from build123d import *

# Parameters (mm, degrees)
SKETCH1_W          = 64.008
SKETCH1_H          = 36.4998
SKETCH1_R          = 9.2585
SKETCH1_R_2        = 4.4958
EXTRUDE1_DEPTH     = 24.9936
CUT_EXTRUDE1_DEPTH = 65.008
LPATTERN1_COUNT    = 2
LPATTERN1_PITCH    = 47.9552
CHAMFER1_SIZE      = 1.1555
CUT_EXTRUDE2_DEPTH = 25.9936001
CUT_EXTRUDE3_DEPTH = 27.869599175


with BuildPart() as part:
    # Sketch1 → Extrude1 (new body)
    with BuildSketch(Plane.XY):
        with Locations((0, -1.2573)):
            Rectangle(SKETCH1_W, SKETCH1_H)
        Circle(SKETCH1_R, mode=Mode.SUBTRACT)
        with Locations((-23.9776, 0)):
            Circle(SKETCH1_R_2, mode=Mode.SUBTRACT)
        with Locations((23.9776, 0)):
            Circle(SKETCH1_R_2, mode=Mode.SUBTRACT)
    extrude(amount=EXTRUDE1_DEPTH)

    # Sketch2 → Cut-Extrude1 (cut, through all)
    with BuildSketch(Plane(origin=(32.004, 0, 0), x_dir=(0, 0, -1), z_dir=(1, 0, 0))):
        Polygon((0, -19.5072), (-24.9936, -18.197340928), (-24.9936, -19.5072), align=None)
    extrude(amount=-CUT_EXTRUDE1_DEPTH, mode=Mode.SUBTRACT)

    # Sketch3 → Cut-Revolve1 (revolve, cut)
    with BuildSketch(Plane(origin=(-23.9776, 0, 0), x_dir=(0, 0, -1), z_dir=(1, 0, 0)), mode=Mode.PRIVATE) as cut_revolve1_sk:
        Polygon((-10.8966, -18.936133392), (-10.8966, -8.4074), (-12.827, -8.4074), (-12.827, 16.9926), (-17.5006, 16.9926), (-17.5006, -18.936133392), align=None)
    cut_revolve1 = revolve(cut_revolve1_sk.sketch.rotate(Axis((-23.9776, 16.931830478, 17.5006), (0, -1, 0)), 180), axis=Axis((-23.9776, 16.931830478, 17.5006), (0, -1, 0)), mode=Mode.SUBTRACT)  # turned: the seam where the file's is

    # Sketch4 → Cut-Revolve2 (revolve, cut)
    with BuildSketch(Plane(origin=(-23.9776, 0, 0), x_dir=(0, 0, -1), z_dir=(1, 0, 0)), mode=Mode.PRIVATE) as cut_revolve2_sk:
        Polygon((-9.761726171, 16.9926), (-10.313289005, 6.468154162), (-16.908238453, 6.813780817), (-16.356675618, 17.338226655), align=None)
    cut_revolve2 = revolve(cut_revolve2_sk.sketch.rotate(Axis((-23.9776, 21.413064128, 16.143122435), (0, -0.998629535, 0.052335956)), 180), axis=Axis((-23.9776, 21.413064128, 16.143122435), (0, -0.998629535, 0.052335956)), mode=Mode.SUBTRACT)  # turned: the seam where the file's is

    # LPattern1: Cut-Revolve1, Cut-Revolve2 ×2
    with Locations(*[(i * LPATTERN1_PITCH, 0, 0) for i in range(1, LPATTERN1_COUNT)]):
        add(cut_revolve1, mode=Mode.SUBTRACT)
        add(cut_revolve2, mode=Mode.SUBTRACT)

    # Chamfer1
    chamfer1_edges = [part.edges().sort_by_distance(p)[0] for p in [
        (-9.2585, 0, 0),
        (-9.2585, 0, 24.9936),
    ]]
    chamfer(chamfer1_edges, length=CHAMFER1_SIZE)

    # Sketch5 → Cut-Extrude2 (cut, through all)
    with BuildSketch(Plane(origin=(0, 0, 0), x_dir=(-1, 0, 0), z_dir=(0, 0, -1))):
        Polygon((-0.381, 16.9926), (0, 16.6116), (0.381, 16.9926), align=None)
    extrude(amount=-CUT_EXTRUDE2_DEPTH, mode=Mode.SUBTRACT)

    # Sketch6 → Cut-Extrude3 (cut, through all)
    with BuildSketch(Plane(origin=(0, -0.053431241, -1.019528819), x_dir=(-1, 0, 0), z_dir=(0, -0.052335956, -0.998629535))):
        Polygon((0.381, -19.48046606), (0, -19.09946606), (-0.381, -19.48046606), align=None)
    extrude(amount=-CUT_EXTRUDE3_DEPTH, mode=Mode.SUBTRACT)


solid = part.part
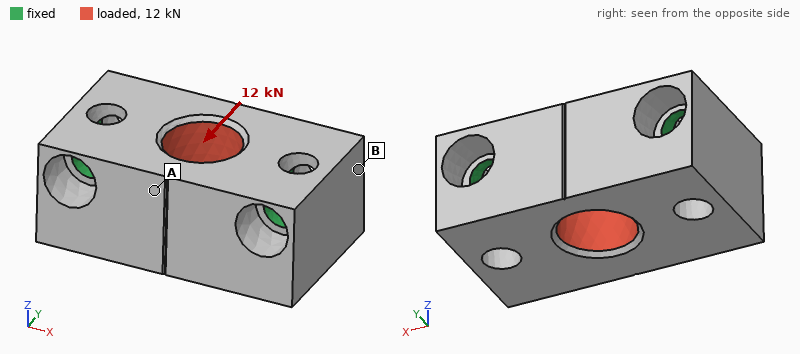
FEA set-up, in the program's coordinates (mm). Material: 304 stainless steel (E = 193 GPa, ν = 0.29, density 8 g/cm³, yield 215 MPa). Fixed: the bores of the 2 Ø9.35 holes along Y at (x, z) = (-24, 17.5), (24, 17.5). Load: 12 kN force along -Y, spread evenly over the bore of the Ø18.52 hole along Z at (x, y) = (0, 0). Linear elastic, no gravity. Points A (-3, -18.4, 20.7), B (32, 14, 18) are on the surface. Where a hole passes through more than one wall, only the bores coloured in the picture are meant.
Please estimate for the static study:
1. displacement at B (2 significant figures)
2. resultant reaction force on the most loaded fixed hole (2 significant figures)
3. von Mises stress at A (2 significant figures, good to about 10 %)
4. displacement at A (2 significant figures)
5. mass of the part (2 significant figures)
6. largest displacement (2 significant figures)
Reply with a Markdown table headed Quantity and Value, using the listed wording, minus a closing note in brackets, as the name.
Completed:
| Quantity | Value |
|---|---|
| displacement at B | 1.9 µm |
| resultant reaction force on the most loaded fixed hole | 6.0 kN |
| von Mises stress at A | 21 MPa |
| displacement at A | 3.6 µm |
| mass of the part | 330 g |
| largest displacement | 7.0 µm |
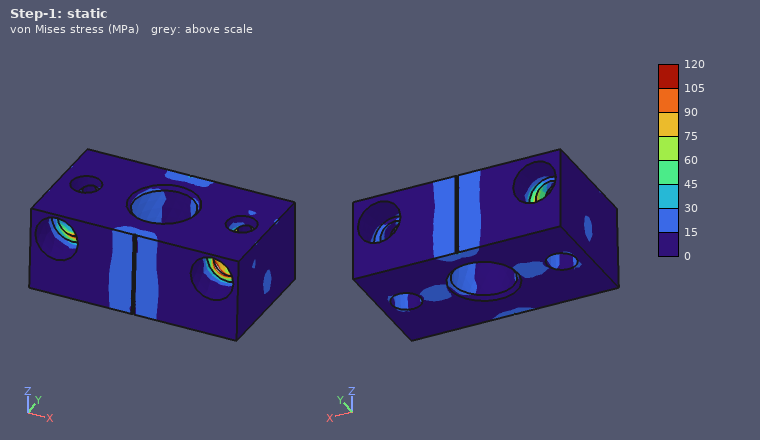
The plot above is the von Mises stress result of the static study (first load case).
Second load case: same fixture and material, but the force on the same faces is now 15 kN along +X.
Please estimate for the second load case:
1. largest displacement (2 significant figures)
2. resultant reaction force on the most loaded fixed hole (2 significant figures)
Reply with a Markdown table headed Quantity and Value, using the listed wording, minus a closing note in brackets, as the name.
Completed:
| Quantity | Value |
|---|---|
| largest displacement | 2.8 µm |
| resultant reaction force on the most loaded fixed hole | 7.6 kN |
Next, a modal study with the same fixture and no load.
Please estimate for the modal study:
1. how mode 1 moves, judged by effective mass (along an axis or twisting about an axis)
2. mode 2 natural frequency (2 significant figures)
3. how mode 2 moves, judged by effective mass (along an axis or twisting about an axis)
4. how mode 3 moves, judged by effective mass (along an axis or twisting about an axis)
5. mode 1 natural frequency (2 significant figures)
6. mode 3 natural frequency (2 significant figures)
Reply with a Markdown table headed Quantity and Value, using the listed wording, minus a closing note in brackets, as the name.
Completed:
| Quantity | Value |
|---|---|
| how mode 1 moves, judged by effective mass | along Y |
| mode 2 natural frequency | 19 kHz |
| how mode 2 moves, judged by effective mass | along Z |
| how mode 3 moves, judged by effective mass | twisting about Z |
| mode 1 natural frequency | 12 kHz |
| mode 3 natural frequency | 21 kHz |
